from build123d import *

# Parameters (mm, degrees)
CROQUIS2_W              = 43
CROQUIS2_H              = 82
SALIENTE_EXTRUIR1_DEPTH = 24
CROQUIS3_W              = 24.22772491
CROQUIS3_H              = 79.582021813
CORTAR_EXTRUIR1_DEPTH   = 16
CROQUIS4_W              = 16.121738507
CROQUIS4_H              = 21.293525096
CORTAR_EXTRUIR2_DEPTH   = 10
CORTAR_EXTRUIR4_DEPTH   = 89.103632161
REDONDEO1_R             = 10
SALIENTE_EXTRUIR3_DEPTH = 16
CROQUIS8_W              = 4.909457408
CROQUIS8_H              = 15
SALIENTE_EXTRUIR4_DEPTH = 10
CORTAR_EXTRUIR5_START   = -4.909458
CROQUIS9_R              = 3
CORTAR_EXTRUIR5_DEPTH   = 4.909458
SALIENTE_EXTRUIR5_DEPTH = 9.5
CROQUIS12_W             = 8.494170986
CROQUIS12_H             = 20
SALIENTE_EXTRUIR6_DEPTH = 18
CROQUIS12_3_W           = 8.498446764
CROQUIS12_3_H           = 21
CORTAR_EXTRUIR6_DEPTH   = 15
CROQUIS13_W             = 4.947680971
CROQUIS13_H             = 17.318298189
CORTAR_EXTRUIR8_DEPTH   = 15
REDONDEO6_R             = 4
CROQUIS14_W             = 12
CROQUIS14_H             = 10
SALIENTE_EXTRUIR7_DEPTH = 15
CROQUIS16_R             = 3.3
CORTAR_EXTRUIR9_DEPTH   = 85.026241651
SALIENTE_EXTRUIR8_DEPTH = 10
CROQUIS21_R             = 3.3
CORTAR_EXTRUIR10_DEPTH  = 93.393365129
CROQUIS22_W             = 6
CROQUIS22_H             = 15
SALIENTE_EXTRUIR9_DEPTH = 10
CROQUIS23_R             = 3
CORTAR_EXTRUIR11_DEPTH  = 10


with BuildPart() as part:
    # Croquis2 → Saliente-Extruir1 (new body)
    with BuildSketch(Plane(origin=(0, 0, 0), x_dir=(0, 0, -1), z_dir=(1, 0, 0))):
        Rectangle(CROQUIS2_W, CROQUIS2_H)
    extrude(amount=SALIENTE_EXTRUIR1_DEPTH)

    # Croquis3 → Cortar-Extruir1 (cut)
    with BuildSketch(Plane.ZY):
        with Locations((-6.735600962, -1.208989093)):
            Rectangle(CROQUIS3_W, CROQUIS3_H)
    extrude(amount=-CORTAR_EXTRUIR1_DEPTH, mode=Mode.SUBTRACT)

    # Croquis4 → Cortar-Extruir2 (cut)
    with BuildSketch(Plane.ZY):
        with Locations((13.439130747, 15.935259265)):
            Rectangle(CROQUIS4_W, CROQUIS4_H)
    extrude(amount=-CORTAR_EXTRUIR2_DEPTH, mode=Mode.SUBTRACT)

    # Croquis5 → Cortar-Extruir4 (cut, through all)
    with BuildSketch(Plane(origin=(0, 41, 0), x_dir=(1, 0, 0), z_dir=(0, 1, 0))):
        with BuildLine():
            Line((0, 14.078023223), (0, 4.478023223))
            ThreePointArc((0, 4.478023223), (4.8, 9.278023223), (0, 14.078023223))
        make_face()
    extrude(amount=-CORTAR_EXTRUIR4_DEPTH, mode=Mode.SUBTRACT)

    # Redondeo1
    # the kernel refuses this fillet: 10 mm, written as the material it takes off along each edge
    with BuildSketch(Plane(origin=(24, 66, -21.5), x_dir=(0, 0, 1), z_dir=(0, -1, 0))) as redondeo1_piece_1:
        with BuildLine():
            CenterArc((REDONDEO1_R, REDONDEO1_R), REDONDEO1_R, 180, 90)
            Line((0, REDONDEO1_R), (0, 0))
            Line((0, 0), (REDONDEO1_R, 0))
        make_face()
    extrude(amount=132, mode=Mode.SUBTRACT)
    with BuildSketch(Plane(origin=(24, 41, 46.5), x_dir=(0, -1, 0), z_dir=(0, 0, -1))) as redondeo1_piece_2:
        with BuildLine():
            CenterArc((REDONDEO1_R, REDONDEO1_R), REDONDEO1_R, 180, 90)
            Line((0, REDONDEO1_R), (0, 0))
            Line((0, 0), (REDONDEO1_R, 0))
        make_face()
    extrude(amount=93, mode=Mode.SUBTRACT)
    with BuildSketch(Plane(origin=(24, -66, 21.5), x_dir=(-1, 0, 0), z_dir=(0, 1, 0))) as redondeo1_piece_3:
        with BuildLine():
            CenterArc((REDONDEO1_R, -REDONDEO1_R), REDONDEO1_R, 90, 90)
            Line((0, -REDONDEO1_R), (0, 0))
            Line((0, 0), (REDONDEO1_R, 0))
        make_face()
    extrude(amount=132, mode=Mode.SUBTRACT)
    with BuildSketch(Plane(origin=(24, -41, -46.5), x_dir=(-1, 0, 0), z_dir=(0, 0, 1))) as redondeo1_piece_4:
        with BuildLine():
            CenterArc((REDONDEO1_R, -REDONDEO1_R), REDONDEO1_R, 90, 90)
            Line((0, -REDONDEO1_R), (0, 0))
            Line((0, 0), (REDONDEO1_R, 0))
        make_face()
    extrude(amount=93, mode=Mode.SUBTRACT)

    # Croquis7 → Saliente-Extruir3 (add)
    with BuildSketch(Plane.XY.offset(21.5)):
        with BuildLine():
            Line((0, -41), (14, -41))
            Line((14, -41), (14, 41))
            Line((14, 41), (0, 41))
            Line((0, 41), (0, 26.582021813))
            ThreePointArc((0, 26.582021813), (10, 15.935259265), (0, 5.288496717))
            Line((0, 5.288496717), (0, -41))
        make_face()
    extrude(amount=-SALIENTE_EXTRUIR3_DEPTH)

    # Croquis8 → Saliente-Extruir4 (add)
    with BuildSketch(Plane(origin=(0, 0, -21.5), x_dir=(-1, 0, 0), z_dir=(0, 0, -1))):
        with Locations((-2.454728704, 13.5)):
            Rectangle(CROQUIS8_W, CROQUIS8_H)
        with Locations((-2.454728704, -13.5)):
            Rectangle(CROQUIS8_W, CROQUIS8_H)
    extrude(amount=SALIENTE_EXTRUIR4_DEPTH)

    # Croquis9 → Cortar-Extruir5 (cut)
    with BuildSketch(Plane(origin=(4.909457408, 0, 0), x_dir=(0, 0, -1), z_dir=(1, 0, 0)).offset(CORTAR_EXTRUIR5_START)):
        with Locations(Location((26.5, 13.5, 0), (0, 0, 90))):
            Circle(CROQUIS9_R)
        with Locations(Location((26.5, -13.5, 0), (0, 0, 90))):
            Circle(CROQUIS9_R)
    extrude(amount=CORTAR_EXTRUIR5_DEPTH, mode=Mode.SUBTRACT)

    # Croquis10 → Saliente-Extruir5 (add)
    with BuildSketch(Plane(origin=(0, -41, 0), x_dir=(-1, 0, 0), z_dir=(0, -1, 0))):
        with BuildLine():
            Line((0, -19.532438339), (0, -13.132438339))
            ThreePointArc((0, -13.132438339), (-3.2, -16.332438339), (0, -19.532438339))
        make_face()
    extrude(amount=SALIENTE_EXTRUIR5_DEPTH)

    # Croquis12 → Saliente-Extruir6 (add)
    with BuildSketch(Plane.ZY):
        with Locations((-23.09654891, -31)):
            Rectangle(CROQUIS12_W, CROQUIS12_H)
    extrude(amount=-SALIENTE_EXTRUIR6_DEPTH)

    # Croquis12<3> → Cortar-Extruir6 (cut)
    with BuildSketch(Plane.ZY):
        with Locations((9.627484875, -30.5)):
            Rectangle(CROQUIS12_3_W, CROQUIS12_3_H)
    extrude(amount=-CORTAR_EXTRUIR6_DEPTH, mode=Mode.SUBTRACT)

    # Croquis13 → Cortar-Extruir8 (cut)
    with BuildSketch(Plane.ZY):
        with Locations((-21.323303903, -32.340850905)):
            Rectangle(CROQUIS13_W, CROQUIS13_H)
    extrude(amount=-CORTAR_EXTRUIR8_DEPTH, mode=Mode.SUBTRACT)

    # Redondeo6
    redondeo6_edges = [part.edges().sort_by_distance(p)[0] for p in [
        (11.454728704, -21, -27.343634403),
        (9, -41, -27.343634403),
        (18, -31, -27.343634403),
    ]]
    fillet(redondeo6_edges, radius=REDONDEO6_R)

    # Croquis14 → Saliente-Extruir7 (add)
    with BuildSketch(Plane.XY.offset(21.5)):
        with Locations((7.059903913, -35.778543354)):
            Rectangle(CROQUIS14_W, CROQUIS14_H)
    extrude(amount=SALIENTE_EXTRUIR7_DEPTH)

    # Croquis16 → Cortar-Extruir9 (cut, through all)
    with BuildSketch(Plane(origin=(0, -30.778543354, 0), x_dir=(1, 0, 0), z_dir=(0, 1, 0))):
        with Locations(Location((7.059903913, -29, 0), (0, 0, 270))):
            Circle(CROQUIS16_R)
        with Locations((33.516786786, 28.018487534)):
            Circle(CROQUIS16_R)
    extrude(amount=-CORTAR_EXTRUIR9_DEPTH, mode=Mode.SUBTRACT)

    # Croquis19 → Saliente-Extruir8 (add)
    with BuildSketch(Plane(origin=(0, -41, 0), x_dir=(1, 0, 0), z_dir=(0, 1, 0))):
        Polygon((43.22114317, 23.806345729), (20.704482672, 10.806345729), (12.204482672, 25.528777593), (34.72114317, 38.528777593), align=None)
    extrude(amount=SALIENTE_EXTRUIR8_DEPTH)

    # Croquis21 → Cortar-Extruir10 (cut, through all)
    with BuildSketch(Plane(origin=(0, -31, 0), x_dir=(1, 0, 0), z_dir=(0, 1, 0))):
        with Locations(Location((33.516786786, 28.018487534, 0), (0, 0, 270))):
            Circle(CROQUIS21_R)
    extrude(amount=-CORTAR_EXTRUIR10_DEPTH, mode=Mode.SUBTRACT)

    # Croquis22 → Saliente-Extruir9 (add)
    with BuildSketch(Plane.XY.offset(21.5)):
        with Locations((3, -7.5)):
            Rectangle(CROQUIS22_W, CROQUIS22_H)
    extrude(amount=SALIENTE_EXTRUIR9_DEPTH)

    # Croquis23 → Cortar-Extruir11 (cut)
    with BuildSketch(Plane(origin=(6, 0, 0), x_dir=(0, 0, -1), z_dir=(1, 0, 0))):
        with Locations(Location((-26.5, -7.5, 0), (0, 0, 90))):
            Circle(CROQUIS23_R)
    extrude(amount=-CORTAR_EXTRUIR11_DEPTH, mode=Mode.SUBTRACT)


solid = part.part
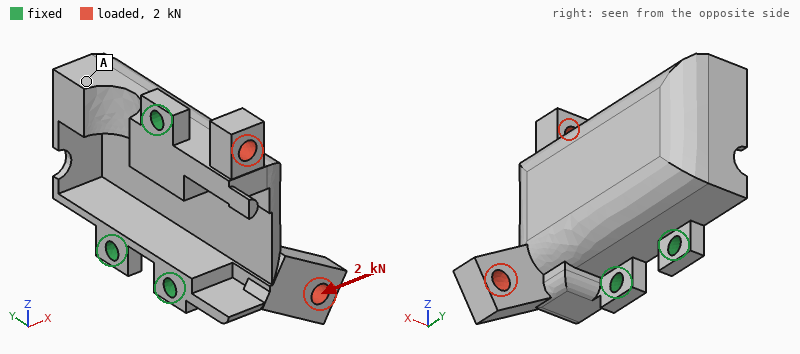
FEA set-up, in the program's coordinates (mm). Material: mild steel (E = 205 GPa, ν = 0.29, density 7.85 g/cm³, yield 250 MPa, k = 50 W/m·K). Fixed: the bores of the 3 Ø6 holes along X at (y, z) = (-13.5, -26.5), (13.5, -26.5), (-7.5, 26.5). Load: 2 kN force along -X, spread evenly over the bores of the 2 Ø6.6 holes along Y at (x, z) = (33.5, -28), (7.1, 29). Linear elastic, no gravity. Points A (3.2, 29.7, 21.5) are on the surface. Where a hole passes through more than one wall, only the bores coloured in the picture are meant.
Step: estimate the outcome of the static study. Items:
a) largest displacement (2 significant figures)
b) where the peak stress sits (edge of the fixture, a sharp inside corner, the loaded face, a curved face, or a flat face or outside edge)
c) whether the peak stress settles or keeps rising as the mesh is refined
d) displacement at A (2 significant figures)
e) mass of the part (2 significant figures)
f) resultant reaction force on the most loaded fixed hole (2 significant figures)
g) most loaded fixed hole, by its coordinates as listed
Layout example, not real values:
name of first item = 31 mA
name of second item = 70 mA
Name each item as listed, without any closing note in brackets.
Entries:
largest displacement = 44 µm
where the peak stress sits = edge of the fixture
whether the peak stress settles or keeps rising as the mesh is refined = keeps rising
displacement at A = 21 µm
mass of the part = 400 g
resultant reaction force on the most loaded fixed hole = 2.1 kN
most loaded fixed hole, by its coordinates as listed = (-13.5, -26.5)
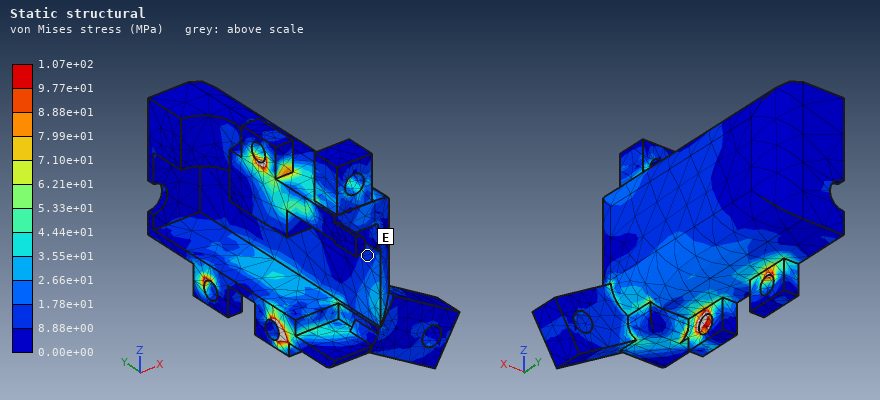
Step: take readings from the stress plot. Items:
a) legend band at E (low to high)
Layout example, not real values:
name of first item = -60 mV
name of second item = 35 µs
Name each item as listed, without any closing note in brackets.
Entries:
legend band at E = 8.88e+00 to 1.78e+01 MPa
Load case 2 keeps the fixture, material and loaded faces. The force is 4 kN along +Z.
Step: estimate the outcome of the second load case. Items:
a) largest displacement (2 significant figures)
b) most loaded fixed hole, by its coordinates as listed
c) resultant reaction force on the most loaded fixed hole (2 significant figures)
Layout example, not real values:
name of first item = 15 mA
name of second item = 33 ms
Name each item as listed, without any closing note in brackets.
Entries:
largest displacement = 56 µm
most loaded fixed hole, by its coordinates as listed = (-7.5, 26.5)
resultant reaction force on the most loaded fixed hole = 4.6 kN
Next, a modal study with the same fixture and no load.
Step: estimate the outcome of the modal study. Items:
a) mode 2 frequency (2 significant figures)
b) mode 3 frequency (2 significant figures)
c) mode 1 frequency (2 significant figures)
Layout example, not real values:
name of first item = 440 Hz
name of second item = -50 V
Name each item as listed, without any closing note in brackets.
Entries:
mode 2 frequency = 4200 Hz
mode 3 frequency = 5600 Hz
mode 1 frequency = 2700 Hz
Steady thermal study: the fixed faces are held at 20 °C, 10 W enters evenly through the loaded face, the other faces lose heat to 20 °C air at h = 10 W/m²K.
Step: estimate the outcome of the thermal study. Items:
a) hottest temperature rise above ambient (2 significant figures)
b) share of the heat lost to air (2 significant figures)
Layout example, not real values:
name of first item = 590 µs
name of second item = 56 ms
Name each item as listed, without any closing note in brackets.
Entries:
hottest temperature rise above ambient = 29 K
share of the heat lost to air = 17 %
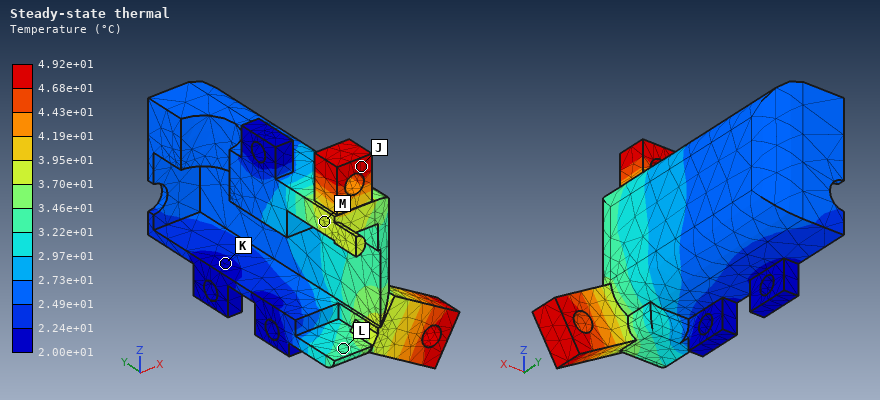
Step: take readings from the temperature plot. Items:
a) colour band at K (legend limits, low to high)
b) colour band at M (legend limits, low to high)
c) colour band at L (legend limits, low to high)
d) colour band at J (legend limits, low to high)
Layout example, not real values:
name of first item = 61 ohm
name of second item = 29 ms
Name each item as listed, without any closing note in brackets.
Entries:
colour band at K = 2.00e+01 to 2.24e+01 °C
colour band at M = 3.70e+01 to 3.95e+01 °C
colour band at L = 3.22e+01 to 3.46e+01 °C
colour band at J = 4.68e+01 to 4.92e+01 °C
